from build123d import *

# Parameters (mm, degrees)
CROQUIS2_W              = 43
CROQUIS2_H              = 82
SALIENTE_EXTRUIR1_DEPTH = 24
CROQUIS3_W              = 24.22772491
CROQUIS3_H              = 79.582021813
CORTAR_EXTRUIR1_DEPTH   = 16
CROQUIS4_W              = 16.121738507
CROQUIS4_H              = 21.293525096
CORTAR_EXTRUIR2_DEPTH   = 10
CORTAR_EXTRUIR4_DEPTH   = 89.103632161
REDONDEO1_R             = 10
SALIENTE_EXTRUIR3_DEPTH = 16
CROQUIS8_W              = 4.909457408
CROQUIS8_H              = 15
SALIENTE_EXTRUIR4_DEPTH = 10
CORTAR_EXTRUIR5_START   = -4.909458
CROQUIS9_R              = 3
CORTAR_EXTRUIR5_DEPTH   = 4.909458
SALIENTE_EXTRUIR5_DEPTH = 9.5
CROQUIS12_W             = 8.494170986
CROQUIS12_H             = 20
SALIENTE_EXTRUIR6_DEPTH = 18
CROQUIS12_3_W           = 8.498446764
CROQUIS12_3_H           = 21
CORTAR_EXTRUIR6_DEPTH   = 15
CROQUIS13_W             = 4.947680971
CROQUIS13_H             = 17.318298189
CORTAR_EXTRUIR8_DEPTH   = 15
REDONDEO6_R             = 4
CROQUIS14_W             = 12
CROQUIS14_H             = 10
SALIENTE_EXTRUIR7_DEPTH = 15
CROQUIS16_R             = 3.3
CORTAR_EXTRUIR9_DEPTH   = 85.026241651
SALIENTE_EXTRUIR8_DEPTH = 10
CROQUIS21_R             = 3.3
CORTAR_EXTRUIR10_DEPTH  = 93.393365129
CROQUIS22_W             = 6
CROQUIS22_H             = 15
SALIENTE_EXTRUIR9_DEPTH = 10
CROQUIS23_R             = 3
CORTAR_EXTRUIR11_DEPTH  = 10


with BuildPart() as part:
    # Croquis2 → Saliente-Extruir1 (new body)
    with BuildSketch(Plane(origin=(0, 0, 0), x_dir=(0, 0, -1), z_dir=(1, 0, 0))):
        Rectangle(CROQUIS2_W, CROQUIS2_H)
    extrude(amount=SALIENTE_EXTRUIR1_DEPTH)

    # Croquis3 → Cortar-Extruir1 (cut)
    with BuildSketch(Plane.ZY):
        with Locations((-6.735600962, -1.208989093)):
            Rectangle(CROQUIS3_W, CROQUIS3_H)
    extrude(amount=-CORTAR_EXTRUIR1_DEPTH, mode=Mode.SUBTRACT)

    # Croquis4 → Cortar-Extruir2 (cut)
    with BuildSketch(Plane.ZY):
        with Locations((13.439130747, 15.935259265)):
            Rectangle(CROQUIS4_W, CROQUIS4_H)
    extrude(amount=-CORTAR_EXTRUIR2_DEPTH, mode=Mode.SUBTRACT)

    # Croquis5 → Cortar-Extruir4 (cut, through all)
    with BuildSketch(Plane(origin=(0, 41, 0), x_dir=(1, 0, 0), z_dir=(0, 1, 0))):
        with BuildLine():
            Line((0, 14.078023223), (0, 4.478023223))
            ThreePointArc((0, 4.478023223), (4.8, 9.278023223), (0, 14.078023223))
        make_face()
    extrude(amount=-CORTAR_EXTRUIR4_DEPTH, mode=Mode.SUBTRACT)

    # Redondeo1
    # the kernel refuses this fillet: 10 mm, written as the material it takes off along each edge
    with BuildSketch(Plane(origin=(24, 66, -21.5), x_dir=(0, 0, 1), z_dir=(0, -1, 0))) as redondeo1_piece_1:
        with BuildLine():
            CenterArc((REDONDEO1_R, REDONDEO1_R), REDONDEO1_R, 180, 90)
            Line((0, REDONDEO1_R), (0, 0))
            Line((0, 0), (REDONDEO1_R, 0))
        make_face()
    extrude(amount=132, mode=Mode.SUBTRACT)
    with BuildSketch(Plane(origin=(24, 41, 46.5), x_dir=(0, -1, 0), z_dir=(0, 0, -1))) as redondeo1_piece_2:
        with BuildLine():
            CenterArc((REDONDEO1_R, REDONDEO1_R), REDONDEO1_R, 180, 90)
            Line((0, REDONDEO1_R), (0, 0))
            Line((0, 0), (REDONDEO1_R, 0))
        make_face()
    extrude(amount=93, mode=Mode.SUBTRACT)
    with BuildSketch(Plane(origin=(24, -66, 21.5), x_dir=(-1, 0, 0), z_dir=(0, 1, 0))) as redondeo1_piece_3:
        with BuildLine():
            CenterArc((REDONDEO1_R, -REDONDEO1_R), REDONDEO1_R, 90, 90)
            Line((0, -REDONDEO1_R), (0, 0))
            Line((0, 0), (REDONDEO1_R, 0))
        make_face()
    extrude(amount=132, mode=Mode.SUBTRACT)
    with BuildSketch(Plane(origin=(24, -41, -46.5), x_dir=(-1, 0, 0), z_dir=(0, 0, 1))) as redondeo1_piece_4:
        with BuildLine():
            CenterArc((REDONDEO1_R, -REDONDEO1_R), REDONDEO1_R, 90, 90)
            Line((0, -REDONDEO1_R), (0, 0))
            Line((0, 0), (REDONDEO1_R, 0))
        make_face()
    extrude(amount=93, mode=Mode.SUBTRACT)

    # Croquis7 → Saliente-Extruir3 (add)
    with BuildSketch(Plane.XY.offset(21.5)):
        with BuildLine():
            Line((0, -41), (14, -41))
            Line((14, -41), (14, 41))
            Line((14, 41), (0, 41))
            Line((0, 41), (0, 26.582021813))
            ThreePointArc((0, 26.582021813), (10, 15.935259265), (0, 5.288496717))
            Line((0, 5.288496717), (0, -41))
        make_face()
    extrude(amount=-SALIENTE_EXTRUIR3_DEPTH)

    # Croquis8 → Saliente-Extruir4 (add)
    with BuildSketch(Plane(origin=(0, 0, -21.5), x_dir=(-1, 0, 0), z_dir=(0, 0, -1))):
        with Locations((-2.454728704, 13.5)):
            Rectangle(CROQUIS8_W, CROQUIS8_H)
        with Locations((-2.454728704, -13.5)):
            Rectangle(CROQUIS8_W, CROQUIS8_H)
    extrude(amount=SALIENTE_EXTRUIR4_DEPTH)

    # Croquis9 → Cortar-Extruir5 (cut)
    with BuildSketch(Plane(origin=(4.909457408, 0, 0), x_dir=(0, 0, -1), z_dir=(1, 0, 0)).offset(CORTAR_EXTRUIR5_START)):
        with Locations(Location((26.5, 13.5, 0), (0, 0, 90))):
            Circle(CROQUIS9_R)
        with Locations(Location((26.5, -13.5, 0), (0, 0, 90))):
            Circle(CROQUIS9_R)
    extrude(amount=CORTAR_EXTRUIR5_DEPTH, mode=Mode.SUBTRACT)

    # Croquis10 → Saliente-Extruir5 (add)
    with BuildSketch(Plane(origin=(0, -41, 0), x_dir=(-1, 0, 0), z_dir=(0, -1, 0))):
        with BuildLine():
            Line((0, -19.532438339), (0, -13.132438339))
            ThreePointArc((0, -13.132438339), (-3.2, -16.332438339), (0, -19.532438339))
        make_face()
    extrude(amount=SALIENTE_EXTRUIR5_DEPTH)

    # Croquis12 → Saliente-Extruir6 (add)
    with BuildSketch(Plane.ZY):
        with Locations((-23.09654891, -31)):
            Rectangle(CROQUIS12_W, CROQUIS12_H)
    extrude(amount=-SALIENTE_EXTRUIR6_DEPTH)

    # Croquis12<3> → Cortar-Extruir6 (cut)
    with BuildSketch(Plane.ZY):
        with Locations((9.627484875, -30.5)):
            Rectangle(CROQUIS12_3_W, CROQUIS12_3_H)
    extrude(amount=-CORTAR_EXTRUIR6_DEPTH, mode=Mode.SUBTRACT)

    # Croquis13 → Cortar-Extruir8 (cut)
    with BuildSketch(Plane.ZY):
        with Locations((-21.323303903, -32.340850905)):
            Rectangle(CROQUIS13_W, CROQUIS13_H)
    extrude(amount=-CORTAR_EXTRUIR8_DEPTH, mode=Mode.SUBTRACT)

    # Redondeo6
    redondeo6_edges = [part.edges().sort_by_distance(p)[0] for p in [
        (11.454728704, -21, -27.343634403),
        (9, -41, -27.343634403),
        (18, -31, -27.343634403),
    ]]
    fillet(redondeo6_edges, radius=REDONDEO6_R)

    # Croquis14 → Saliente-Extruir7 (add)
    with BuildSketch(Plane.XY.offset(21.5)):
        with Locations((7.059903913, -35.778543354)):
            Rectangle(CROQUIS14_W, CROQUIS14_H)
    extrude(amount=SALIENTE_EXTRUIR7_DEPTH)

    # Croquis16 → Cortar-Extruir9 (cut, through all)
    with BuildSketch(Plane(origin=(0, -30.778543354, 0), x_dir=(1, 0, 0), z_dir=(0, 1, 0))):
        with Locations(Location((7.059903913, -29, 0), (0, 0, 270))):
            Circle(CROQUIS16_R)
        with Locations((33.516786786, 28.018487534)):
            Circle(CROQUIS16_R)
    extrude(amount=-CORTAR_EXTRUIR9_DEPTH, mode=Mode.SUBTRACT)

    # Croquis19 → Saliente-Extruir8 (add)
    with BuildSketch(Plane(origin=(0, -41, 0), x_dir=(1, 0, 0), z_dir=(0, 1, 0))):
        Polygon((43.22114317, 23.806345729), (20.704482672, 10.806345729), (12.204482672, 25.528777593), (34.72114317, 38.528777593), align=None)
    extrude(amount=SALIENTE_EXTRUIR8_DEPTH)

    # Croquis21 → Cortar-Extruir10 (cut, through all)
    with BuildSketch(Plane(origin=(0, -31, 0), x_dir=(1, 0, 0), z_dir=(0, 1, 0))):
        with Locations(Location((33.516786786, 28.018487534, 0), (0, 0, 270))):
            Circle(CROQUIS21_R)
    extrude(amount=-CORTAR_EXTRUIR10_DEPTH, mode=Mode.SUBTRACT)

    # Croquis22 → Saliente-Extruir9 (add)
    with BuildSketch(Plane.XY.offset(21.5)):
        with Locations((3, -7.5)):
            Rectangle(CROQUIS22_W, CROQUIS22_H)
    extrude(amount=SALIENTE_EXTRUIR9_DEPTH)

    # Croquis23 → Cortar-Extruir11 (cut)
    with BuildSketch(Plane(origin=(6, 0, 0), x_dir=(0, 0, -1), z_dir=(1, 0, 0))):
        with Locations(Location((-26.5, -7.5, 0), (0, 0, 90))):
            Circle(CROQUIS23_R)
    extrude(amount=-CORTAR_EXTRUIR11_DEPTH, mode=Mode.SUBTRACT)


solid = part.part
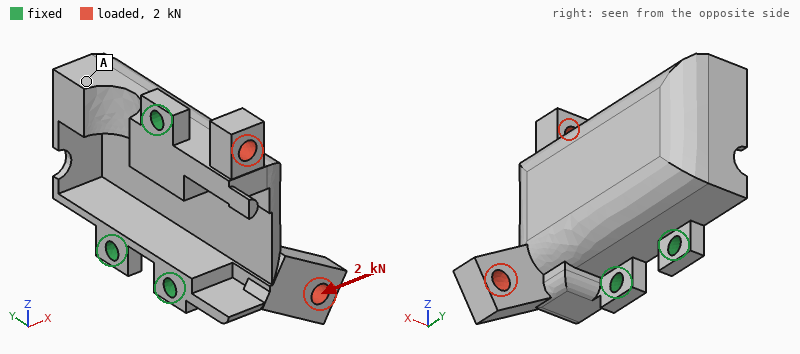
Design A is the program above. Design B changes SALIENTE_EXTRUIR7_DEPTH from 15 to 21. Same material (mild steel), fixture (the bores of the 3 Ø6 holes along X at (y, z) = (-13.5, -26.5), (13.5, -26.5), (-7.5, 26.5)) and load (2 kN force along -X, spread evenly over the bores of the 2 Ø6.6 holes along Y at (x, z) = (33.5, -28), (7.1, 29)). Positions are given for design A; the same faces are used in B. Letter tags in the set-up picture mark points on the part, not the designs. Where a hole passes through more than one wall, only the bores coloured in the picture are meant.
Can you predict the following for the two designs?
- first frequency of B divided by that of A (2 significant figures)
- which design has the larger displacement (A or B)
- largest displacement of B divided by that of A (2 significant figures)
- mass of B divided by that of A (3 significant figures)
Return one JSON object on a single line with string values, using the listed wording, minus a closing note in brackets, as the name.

{"first frequency of B divided by that of A": "0.99", "which design has the larger displacement": "B", "largest displacement of B divided by that of A": "1.1", "mass of B divided by that of A": "1.01"}
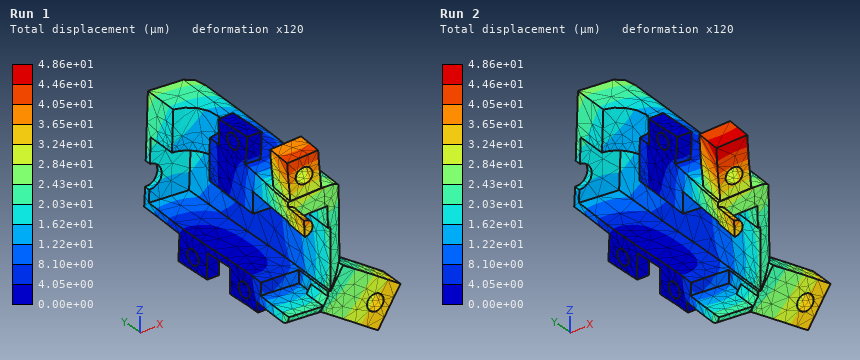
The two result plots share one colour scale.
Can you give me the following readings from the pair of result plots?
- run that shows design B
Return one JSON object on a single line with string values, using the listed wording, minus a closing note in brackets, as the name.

{"run that shows design B": "Run 2"}
